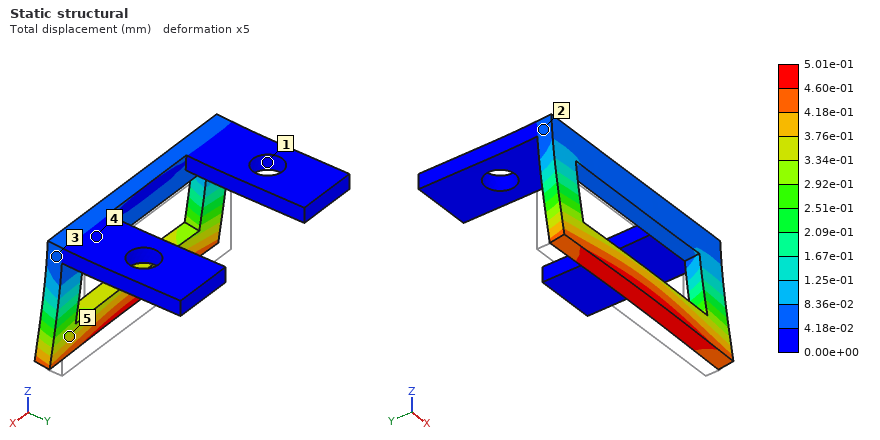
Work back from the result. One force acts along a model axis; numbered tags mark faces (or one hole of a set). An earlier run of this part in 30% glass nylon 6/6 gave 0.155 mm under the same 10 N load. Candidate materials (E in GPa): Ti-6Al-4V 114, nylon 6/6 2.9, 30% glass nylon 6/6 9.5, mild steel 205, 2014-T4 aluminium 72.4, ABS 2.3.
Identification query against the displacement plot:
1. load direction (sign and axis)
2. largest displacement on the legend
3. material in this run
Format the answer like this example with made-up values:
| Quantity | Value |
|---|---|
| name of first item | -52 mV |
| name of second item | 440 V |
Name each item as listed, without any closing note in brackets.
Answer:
| Quantity | Value |
|---|---|
| load direction | -Y |
| largest displacement on the legend | 5.01e-01 mm |
| material in this run | nylon 6/6 |
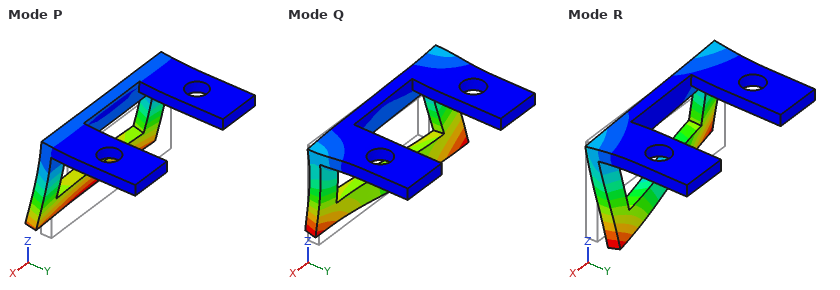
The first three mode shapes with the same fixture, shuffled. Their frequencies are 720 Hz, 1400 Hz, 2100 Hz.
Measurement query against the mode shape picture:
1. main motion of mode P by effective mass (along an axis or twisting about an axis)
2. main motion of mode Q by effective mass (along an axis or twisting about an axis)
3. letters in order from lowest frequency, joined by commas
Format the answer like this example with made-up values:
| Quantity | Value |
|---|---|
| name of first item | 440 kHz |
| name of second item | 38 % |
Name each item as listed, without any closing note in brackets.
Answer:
| Quantity | Value |
|---|---|
| main motion of mode P by effective mass | along Y |
| main motion of mode Q by effective mass | along X |
| letters in order from lowest frequency, joined by commas | P, R, Q |
